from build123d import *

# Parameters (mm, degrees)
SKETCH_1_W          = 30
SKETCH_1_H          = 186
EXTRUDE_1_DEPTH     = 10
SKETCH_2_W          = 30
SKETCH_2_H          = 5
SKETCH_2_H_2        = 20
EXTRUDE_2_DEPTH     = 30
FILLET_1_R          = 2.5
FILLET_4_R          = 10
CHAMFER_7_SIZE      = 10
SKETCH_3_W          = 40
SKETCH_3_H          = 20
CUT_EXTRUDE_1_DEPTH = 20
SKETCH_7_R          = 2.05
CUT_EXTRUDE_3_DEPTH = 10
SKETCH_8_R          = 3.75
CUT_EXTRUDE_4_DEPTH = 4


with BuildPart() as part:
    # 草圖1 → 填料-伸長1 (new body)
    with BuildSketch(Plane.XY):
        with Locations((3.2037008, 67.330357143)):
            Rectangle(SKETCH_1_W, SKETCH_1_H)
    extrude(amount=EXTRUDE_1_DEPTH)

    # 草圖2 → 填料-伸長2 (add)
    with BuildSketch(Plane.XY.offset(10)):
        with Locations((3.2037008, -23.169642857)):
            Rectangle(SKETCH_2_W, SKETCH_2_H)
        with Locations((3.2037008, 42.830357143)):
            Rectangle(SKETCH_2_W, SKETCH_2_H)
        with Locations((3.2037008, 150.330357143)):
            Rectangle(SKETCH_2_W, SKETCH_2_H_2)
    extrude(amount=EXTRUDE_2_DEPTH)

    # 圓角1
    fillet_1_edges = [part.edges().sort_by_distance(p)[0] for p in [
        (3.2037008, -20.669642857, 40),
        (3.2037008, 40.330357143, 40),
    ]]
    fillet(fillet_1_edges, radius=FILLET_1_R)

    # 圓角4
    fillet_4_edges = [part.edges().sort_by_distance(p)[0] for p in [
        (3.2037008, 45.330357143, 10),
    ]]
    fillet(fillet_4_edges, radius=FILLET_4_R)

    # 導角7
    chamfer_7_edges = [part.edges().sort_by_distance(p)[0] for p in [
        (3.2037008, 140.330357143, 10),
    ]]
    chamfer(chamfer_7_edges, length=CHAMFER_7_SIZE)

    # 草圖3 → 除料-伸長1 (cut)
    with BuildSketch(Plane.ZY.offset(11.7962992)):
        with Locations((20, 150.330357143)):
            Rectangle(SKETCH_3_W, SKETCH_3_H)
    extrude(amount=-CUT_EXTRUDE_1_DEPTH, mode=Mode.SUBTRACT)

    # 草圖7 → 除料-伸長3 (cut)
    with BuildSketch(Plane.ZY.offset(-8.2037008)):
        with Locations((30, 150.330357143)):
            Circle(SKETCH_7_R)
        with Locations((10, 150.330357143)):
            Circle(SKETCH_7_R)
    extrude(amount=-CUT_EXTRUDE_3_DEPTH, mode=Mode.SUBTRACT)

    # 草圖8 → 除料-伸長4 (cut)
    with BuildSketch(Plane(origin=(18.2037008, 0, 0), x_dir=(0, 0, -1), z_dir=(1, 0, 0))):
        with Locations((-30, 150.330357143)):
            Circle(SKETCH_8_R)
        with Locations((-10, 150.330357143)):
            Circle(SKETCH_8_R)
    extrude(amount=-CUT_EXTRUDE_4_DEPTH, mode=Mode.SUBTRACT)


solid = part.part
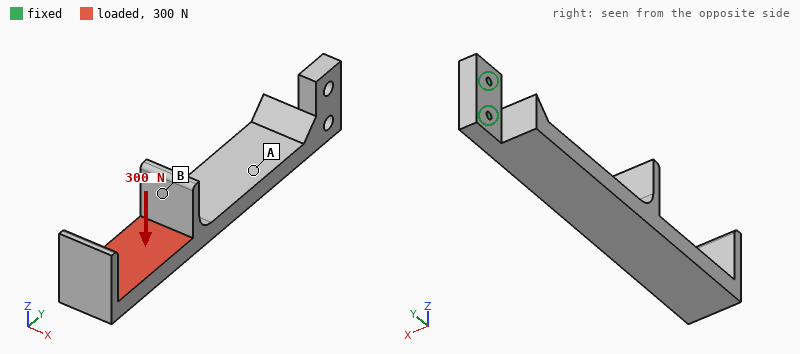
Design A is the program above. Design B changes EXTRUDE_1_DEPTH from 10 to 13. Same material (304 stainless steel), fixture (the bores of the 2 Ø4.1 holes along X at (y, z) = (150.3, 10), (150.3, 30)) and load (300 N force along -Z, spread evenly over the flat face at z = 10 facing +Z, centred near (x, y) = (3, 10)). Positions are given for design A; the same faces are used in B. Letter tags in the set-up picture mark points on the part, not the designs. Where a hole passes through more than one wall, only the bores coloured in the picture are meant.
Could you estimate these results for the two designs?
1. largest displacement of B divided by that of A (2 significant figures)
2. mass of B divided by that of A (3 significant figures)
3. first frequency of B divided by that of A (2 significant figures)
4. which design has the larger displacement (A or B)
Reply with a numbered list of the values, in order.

1. 0.51
2. 1.21
3. 1.0
4. A
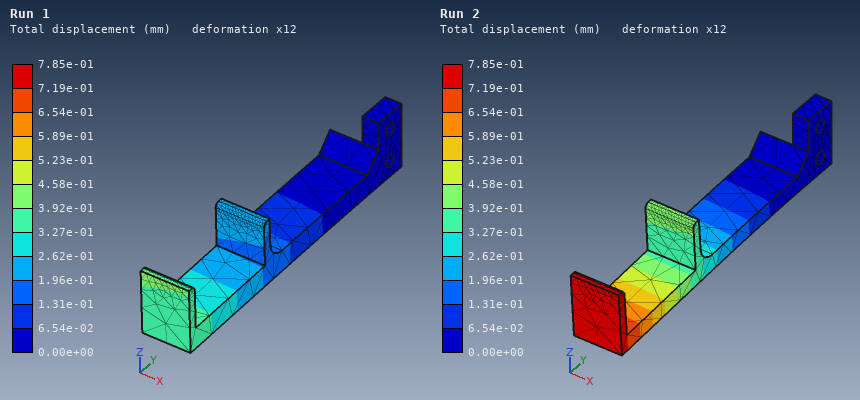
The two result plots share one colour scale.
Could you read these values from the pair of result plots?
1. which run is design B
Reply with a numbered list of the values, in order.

1. Run 1
